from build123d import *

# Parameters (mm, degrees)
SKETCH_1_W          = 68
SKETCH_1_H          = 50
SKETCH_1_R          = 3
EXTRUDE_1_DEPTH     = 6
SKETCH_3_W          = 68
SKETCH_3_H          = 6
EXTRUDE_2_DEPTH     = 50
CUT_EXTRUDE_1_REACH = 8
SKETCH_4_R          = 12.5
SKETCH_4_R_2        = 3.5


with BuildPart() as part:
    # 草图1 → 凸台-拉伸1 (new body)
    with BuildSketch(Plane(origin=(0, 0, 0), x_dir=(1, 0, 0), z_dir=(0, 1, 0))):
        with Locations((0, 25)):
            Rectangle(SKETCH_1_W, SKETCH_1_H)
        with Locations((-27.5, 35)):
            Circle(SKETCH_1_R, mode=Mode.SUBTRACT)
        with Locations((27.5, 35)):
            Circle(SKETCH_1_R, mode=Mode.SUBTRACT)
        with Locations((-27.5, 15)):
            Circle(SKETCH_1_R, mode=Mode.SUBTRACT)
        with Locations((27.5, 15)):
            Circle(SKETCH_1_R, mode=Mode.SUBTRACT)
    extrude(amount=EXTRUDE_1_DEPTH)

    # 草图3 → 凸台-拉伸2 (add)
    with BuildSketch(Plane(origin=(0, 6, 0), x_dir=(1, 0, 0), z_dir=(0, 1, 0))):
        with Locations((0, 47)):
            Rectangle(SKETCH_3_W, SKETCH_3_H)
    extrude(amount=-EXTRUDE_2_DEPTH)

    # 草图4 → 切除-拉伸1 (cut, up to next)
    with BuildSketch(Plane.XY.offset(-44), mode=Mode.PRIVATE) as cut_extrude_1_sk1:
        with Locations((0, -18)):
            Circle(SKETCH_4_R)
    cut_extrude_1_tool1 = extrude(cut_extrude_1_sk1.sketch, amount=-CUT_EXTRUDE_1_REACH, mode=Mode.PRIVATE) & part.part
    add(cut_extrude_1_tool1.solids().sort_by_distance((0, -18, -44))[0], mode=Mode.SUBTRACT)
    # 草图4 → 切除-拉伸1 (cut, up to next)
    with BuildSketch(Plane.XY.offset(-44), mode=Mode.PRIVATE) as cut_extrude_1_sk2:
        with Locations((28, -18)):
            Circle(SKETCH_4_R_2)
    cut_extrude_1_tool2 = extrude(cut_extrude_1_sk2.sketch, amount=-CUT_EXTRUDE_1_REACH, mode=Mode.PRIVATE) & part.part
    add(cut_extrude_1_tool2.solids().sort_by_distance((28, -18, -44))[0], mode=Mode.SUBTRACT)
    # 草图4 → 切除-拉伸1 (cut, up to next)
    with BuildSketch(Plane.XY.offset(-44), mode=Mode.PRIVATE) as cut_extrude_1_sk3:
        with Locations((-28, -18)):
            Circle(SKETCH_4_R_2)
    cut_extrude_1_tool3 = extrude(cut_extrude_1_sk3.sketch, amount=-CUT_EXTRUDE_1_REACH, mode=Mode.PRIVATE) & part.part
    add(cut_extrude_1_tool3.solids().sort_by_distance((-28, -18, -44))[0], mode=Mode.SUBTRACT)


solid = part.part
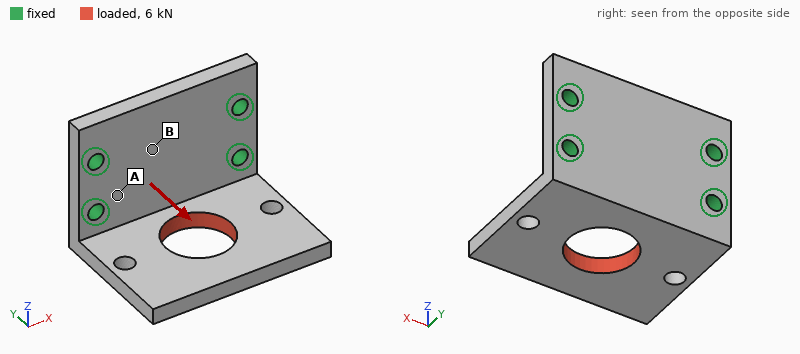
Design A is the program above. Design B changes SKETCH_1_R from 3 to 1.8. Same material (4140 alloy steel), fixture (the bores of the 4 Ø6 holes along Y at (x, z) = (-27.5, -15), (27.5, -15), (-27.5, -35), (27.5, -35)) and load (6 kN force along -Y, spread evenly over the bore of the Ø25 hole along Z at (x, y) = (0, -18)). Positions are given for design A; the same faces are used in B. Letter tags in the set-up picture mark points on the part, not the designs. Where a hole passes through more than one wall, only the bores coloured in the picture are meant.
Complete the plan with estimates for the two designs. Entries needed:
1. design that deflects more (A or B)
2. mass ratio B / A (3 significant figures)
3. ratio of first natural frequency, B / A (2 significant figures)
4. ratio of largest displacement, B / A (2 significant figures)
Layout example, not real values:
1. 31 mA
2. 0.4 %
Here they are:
1. B
2. 1.01
3. 0.97
4. 1.3
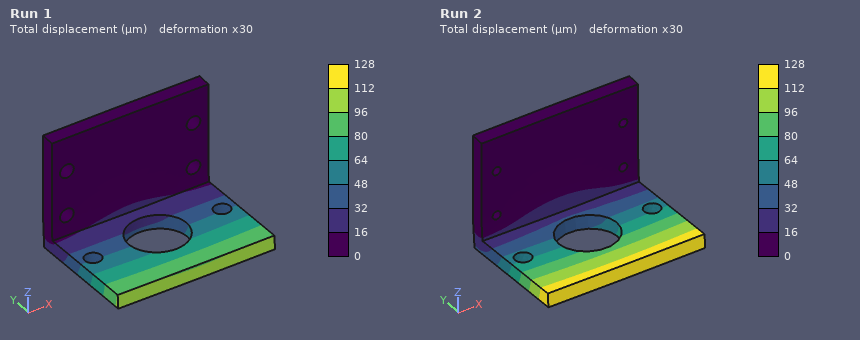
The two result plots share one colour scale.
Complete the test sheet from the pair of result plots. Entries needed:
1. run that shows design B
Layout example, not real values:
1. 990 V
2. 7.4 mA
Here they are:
1. Run 2
